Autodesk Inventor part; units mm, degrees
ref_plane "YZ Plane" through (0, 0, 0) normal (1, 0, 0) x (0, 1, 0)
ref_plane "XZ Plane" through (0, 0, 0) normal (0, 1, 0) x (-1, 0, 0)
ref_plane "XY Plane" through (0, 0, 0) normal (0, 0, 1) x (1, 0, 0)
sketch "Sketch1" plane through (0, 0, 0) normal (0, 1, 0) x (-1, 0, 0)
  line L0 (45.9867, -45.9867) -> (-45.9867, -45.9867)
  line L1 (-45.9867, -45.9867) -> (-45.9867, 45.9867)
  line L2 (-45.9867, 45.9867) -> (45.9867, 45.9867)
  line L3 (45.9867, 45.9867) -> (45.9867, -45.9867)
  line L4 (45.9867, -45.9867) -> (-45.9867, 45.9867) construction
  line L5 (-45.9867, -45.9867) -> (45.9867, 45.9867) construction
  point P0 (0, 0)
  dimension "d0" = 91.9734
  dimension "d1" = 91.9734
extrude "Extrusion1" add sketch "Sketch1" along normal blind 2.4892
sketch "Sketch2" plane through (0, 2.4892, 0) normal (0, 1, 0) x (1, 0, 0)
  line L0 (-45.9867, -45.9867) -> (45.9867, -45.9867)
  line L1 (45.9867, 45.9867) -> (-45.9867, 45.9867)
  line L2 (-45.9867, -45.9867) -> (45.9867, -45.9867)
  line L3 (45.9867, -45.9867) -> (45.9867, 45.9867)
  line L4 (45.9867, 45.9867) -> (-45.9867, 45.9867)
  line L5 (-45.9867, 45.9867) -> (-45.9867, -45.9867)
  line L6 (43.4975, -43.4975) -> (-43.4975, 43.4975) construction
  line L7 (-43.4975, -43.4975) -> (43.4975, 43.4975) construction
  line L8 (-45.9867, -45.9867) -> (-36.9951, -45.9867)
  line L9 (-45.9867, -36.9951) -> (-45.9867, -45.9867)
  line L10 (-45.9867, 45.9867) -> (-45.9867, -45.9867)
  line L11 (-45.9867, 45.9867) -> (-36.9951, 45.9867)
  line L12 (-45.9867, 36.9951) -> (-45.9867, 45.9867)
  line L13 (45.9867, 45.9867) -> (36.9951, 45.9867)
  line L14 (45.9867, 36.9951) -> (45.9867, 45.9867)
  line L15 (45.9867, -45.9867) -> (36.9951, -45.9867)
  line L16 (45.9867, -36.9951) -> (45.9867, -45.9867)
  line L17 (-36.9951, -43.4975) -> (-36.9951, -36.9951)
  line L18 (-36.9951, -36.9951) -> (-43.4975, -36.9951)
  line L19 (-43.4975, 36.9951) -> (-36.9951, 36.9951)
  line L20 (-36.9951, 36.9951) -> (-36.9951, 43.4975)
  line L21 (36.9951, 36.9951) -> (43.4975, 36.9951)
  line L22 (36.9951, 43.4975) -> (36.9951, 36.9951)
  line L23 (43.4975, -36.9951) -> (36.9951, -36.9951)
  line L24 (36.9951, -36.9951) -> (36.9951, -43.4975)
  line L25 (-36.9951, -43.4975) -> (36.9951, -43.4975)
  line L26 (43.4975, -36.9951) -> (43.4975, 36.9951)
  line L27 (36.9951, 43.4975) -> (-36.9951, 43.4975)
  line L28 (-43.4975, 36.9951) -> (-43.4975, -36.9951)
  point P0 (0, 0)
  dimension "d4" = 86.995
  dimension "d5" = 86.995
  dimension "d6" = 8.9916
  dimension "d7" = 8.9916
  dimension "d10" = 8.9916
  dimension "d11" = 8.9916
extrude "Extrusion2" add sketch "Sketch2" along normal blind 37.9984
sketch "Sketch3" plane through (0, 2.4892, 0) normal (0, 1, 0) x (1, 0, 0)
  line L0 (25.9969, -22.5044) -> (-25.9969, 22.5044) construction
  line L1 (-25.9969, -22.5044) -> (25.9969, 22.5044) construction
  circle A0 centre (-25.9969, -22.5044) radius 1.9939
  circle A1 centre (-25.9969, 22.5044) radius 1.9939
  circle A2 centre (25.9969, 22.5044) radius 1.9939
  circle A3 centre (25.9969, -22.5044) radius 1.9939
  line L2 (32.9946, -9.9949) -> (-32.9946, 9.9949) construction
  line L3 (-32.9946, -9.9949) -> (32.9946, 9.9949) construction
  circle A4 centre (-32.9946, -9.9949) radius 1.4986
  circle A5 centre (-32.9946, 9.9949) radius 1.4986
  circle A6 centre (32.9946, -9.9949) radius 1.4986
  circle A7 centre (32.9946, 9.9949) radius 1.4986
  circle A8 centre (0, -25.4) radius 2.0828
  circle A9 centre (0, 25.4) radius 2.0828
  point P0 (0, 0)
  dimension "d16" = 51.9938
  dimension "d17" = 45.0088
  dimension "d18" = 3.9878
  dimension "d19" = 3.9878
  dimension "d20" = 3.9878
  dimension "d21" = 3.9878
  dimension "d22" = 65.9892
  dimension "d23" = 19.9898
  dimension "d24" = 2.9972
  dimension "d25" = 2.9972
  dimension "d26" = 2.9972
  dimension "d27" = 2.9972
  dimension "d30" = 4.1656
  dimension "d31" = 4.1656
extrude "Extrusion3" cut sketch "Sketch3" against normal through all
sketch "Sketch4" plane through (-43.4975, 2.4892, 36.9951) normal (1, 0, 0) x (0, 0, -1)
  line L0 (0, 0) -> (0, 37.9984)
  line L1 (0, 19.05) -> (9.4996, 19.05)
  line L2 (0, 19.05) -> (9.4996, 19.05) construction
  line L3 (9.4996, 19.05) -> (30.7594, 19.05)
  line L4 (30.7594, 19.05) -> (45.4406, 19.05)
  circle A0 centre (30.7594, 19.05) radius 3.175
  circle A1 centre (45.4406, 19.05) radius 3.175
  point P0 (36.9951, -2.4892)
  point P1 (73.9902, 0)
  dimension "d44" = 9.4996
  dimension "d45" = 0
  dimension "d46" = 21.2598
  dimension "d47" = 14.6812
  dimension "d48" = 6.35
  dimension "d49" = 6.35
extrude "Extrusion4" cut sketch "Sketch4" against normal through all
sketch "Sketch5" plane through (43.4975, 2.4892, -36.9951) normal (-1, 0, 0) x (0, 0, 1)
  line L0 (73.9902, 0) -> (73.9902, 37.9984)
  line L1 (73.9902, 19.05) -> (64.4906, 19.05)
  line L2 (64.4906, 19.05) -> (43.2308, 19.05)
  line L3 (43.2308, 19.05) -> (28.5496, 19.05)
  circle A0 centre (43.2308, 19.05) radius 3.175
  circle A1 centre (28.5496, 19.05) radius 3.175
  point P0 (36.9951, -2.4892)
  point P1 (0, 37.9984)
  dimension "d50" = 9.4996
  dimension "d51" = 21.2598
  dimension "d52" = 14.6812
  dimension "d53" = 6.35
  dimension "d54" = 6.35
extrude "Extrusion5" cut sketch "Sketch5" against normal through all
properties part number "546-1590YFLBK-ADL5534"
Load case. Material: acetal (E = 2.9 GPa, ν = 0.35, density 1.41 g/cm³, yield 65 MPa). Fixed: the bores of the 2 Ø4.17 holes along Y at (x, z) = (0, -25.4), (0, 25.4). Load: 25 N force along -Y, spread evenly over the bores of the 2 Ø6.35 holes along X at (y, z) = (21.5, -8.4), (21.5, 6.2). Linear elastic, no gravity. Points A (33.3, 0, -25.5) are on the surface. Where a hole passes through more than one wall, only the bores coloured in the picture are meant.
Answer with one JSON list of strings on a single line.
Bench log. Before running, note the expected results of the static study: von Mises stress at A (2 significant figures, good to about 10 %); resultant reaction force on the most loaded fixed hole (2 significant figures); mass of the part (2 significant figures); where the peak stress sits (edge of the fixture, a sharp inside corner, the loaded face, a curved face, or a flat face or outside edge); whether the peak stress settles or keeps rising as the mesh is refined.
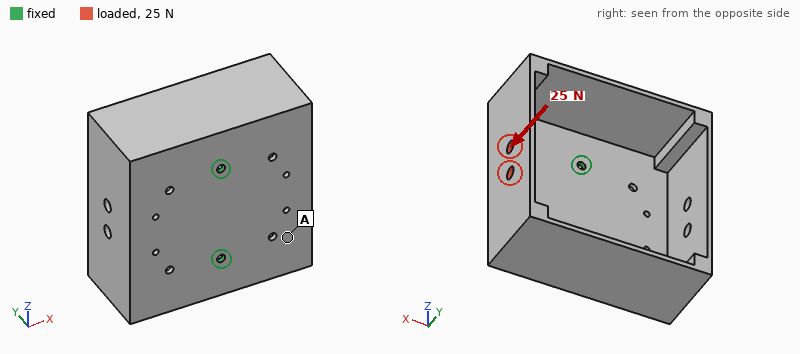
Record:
["1.2 MPa", "13 N", "86 g", "edge of the fixture", "keeps rising"]
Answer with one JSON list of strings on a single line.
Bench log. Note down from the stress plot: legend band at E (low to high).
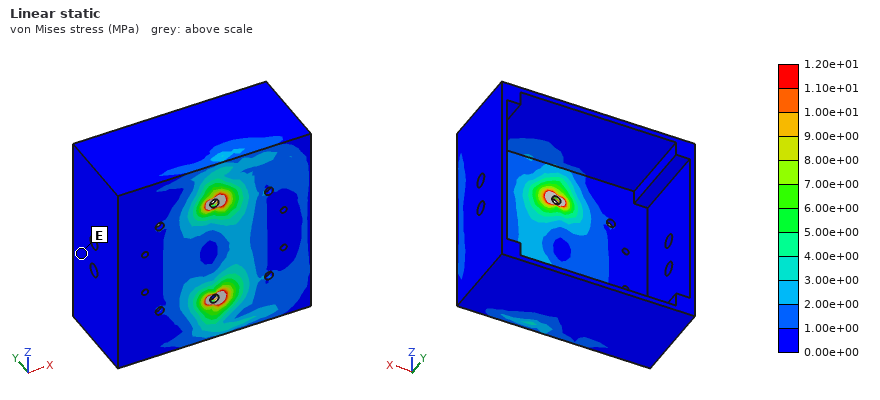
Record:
["0.00e+00 to 1.00e+00 MPa"]
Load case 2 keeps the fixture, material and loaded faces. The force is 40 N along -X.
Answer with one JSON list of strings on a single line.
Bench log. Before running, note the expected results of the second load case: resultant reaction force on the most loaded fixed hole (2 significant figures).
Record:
["22 N"]
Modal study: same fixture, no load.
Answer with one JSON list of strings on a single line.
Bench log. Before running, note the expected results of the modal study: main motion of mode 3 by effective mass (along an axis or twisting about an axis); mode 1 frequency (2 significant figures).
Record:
["along Z", "97 Hz"]
